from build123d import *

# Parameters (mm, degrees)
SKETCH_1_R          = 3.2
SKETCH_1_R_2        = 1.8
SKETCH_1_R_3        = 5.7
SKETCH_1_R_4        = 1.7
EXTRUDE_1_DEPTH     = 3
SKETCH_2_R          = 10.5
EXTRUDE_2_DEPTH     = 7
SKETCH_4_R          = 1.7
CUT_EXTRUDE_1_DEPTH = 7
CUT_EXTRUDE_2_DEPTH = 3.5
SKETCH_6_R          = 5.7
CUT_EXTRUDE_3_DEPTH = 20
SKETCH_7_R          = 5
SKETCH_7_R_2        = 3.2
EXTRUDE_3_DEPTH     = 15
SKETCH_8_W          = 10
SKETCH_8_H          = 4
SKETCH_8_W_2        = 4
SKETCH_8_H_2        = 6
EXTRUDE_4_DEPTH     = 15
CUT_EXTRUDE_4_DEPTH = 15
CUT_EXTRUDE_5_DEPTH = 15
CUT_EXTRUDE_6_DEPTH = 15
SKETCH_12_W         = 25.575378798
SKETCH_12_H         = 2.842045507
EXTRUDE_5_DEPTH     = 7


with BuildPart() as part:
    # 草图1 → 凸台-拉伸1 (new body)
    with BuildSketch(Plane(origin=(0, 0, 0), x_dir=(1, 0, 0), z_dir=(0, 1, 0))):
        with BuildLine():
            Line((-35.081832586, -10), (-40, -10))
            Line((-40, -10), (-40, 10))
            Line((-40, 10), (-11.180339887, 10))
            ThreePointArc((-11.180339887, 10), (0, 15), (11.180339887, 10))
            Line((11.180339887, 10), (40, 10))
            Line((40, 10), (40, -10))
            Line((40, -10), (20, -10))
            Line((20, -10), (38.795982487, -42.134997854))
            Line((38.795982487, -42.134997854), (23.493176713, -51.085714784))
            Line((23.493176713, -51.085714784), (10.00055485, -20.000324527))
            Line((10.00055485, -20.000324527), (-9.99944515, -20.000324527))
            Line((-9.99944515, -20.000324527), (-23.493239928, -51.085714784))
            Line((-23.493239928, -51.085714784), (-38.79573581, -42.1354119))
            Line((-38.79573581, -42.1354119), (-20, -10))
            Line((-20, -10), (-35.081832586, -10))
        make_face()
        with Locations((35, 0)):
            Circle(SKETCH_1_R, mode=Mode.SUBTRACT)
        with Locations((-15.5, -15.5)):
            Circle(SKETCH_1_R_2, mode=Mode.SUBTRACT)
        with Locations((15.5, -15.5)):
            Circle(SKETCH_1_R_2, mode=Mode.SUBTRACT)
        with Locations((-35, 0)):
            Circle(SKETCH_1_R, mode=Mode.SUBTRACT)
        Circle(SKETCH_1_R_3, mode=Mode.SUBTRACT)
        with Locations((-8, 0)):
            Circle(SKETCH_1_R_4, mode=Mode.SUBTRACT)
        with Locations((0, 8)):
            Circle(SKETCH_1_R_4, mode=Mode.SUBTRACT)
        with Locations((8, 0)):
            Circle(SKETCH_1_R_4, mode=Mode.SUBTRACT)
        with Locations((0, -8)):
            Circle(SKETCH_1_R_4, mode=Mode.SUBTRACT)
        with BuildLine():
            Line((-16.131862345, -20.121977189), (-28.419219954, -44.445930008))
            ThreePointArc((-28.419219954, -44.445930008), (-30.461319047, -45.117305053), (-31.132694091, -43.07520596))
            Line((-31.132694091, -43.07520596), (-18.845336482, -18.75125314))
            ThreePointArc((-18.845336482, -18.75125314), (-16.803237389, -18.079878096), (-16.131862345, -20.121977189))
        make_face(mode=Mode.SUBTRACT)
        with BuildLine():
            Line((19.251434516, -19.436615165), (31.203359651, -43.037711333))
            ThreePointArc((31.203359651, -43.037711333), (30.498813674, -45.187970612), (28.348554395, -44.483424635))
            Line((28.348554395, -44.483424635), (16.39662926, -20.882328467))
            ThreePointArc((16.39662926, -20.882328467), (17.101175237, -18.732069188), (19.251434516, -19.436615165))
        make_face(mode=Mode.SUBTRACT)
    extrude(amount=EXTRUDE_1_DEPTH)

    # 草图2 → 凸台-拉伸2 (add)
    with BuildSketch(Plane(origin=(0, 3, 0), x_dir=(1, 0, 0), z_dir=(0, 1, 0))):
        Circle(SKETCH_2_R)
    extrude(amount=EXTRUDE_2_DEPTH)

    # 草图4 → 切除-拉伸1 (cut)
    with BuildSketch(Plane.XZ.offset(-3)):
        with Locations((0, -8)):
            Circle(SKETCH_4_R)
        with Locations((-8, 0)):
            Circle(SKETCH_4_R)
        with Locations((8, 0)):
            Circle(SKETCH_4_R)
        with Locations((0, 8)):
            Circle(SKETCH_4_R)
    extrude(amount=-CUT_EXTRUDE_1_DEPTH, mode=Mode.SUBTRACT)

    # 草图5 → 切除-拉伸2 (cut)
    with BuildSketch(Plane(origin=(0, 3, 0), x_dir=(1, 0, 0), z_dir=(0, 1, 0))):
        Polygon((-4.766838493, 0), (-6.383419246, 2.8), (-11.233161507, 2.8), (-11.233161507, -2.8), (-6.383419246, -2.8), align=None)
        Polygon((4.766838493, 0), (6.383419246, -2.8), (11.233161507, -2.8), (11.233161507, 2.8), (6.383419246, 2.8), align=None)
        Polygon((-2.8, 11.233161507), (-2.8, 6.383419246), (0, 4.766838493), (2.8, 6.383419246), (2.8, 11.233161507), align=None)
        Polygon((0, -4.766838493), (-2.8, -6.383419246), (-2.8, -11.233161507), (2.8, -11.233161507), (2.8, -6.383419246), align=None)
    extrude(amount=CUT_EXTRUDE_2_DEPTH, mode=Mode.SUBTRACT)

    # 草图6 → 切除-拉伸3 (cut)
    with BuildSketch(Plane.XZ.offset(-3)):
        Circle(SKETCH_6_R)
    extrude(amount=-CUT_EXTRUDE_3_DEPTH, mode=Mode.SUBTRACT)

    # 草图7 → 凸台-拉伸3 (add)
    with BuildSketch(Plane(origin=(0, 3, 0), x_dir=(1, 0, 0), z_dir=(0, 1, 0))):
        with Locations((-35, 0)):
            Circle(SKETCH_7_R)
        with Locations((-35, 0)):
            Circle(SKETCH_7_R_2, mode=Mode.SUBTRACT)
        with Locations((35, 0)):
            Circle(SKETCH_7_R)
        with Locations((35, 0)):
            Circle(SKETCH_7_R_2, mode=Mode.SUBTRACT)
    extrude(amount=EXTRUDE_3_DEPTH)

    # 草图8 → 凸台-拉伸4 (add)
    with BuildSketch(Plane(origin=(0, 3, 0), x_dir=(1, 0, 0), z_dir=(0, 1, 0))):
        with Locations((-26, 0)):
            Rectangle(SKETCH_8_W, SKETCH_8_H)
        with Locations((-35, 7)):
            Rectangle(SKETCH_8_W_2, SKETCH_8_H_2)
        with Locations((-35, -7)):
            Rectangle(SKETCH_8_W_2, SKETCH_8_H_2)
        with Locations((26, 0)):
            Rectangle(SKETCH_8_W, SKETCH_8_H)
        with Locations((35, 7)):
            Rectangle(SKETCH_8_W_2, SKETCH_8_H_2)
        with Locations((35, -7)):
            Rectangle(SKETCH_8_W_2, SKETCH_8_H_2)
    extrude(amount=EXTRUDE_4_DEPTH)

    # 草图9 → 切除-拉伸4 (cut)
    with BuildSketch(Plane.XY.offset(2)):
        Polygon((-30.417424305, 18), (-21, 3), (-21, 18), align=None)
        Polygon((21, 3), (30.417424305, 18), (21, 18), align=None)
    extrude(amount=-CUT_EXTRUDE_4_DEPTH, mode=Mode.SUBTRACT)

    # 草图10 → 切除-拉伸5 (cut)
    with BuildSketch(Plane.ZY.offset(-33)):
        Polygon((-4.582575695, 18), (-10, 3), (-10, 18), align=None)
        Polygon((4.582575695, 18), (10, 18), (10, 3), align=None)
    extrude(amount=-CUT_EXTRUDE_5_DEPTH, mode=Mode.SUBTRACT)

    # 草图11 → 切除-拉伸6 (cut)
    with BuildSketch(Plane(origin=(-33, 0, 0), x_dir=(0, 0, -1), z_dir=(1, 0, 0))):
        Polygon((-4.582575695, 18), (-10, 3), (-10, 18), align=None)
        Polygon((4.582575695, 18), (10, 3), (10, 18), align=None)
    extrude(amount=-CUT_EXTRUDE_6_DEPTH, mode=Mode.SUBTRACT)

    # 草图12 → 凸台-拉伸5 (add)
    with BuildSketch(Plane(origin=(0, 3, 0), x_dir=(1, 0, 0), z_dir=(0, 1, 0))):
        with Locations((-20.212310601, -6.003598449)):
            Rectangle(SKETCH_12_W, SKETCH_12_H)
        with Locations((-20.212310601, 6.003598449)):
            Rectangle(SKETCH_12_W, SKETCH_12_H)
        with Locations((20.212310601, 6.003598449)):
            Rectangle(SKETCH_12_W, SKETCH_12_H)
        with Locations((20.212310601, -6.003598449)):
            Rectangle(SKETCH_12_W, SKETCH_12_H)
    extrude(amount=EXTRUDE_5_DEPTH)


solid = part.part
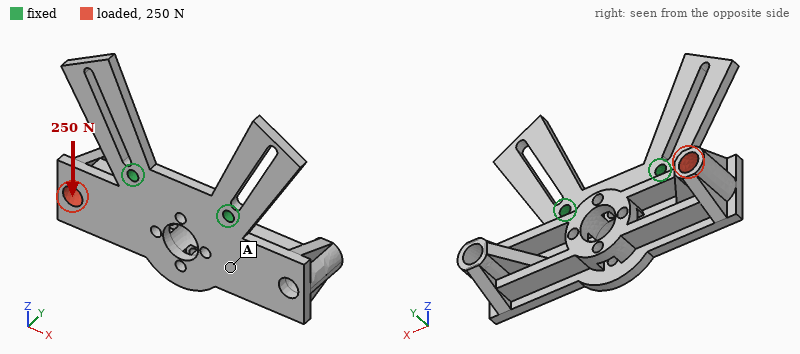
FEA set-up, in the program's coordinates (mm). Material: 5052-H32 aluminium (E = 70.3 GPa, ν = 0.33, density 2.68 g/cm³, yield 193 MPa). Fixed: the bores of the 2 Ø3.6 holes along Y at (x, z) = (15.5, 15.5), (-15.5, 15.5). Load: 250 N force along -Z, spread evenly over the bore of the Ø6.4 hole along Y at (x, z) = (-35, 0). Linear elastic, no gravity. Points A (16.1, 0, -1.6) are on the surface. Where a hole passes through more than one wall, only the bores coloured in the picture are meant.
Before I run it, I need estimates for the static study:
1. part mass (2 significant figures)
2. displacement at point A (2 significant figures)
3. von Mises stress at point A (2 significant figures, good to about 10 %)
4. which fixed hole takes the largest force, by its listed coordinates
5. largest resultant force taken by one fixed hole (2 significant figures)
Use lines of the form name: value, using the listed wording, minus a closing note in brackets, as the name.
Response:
part mass: 37 g
displacement at point A: 0.028 mm
von Mises stress at point A: 8.0 MPa
which fixed hole takes the largest force, by its listed coordinates: (-15.5, 15.5)
largest resultant force taken by one fixed hole: 400 N
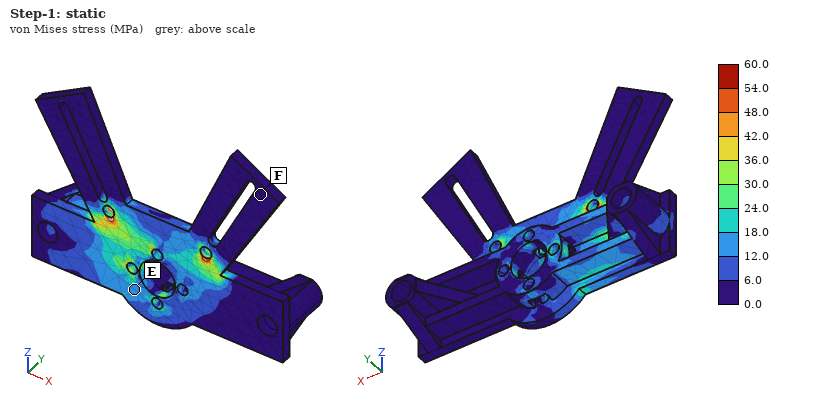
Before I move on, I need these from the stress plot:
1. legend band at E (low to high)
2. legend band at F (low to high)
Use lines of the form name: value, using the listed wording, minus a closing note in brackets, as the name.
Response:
legend band at E: 12.0 to 18.0 MPa
legend band at F: 0.0 to 6.0 MPa
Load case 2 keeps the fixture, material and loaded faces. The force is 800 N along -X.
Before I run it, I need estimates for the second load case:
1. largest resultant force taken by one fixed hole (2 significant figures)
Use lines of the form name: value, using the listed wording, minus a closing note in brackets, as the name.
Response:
largest resultant force taken by one fixed hole: 570 N
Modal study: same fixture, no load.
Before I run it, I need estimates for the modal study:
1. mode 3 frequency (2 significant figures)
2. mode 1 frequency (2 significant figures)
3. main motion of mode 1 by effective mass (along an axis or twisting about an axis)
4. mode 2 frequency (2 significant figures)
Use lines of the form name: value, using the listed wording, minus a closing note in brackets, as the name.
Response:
mode 3 frequency: 1900 Hz
mode 1 frequency: 1700 Hz
main motion of mode 1 by effective mass: along Y
mode 2 frequency: 1900 Hz
